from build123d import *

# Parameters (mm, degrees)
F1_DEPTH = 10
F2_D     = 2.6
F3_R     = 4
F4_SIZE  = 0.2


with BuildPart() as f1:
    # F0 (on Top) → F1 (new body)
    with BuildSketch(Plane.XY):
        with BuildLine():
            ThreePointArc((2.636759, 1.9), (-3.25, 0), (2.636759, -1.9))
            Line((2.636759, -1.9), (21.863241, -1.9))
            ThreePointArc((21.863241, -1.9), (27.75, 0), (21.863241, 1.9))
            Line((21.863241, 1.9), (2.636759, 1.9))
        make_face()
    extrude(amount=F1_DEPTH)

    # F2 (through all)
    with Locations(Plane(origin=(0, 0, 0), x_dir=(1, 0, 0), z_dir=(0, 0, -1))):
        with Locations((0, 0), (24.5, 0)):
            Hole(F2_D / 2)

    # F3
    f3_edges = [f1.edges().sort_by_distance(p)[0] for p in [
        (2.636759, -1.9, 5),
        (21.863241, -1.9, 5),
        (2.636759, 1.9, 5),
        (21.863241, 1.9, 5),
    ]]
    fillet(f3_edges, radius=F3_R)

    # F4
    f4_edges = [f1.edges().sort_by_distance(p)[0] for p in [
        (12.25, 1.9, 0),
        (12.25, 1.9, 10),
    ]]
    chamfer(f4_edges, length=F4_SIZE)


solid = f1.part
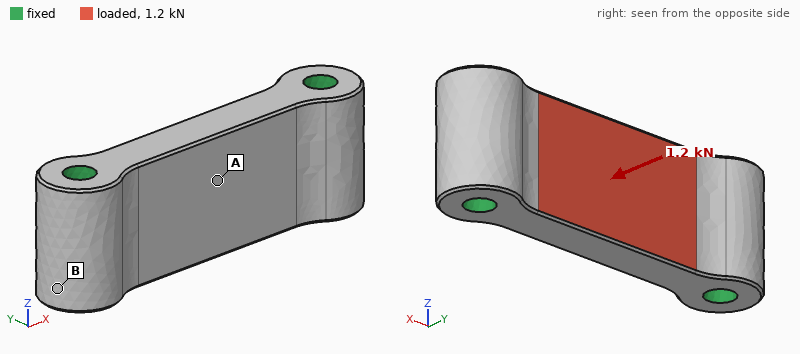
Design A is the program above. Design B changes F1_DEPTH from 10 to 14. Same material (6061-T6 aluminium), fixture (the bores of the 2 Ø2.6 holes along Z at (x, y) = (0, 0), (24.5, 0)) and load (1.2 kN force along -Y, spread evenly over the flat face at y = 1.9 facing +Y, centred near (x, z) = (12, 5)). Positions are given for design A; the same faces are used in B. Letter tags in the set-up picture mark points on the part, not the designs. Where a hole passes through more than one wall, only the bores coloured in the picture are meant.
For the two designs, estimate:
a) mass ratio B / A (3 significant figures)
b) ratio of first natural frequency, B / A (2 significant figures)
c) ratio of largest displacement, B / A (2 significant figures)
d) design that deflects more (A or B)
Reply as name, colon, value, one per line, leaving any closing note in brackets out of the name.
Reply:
mass ratio B / A: 1.40
ratio of first natural frequency, B / A: 1.0
ratio of largest displacement, B / A: 0.72
design that deflects more: A
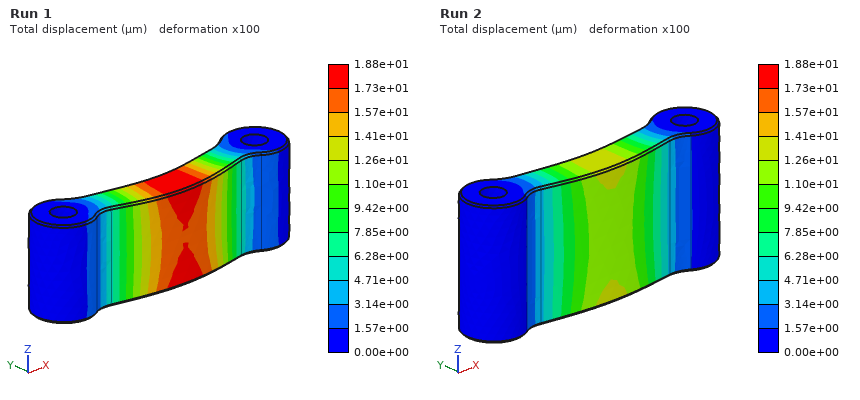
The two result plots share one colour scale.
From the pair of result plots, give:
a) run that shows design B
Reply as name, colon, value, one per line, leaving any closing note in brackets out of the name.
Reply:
run that shows design B: Run 2
